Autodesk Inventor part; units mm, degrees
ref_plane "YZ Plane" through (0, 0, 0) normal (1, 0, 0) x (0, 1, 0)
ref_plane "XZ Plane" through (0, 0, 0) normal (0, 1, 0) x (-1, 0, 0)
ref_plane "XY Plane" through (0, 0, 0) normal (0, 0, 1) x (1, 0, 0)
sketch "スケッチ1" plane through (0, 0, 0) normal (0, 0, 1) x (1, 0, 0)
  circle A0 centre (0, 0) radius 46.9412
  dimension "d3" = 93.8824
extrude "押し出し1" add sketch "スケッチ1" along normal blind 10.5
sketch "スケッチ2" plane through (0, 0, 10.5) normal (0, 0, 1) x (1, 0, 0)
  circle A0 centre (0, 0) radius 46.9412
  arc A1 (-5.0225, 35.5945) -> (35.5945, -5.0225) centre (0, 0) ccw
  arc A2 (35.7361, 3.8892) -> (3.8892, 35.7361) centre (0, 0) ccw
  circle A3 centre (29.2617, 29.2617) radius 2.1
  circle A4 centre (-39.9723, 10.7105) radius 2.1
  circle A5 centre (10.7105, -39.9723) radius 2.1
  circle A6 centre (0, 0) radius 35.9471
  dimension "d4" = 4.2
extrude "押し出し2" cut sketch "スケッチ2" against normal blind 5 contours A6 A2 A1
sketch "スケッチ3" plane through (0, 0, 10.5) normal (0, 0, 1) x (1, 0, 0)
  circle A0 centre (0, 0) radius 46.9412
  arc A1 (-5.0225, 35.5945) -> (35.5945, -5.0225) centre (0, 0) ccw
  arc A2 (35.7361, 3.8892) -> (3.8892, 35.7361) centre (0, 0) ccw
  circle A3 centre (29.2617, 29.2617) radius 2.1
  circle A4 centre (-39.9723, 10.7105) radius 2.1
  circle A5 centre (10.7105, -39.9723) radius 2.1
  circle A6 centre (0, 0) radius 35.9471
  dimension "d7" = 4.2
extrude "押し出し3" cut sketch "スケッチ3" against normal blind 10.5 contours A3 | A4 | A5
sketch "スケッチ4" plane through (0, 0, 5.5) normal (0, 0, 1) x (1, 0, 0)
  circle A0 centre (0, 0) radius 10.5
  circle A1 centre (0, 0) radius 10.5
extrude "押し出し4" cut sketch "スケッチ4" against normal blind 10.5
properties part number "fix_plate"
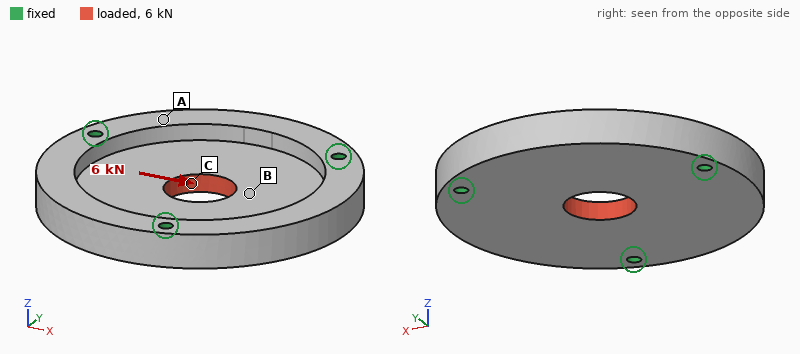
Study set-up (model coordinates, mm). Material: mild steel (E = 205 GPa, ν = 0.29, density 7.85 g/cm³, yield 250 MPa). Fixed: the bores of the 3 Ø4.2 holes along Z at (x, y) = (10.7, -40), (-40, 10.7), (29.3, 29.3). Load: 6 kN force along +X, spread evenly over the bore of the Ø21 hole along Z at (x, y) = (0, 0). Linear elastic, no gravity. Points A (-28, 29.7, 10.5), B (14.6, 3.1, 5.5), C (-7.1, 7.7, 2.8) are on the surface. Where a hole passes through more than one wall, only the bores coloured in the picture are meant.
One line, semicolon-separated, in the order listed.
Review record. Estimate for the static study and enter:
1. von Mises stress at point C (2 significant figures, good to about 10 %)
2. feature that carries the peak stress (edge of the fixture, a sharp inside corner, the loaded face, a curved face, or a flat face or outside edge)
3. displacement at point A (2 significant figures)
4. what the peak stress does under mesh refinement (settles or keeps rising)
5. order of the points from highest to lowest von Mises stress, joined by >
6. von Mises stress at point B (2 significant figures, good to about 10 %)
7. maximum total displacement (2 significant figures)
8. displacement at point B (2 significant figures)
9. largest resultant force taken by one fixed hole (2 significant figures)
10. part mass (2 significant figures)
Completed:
25 MPa; edge of the fixture; 0.96 µm; keeps rising; C > B > A; 16 MPa; 3.9 µm; 3.3 µm; 2.0 kN; 390 g
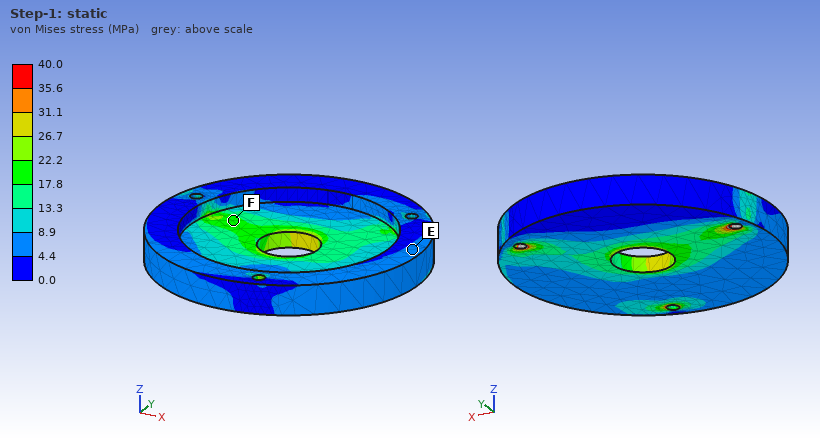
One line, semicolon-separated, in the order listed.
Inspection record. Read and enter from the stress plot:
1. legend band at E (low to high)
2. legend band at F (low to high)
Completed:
4.4 to 8.9 MPa; 17.8 to 22.2 MPa
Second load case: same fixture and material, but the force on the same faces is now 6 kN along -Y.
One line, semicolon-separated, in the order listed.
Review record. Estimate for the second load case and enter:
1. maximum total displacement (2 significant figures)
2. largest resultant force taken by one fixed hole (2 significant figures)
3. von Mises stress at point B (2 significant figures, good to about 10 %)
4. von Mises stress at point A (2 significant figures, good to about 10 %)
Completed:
3.9 µm; 2.0 kN; 18 MPa; 5.7 MPa
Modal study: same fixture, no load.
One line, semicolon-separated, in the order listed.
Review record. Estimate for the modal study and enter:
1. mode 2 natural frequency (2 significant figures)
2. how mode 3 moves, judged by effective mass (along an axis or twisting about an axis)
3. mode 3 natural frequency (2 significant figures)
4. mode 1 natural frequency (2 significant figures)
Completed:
5900 Hz; along Z; 6200 Hz; 5900 Hz
